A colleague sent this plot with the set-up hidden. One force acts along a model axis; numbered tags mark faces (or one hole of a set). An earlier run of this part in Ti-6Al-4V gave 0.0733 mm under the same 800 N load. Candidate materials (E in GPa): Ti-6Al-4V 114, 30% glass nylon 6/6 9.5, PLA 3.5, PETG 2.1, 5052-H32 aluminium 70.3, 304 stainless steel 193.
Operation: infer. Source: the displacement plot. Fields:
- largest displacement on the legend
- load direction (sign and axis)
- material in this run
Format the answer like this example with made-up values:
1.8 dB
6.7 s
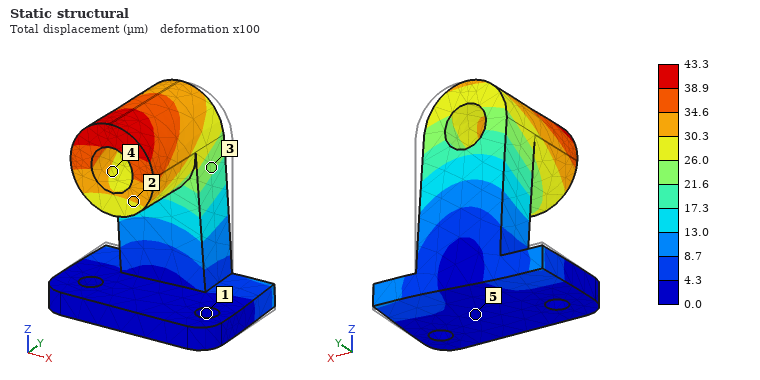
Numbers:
43.3 µm
-X
304 stainless steel
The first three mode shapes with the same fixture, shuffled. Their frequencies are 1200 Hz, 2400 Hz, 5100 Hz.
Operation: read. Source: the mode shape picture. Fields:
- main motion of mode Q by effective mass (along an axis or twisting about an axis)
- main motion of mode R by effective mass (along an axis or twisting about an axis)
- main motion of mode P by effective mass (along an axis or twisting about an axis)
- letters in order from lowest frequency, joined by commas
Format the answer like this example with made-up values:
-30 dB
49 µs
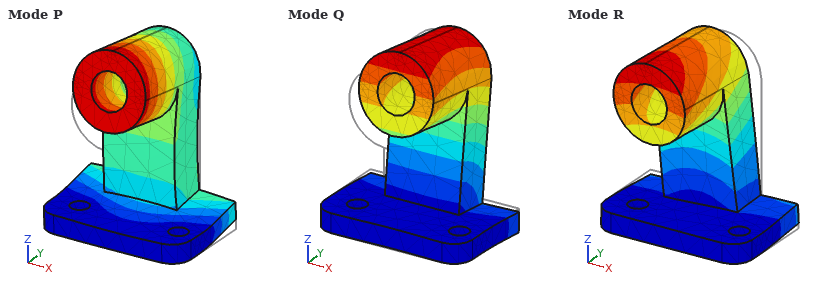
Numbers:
along Y
along X
along Z
Q, R, P
